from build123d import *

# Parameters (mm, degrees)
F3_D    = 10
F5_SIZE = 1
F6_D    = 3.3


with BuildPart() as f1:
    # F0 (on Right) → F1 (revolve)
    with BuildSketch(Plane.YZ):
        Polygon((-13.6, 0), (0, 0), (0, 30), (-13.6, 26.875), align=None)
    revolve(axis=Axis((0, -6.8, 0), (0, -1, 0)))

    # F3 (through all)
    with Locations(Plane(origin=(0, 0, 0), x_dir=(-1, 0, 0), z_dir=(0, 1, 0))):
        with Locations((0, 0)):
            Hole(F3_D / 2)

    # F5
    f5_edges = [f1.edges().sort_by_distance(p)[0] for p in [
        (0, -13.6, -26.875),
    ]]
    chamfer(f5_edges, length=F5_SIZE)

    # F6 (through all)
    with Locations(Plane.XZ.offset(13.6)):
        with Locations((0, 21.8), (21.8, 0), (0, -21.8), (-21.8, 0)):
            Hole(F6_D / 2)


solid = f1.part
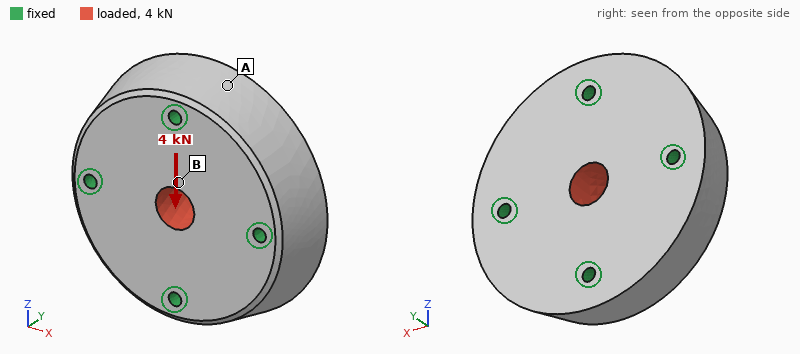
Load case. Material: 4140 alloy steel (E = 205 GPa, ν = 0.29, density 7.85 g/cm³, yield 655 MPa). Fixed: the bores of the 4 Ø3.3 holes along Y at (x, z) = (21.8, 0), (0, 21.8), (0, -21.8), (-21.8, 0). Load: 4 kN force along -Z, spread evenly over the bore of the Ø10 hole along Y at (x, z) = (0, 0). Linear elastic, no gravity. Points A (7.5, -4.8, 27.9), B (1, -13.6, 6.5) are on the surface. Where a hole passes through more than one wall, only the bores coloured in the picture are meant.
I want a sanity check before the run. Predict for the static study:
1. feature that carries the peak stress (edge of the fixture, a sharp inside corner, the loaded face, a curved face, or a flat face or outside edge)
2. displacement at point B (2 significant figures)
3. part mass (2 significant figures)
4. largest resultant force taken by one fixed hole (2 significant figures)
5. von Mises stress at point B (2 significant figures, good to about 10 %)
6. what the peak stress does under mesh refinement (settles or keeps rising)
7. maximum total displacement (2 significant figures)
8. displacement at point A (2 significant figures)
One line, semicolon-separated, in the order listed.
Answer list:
edge of the fixture; 0.66 µm; 260 g; 1.3 kN; 10 MPa; keeps rising; 0.78 µm; 0.18 µm
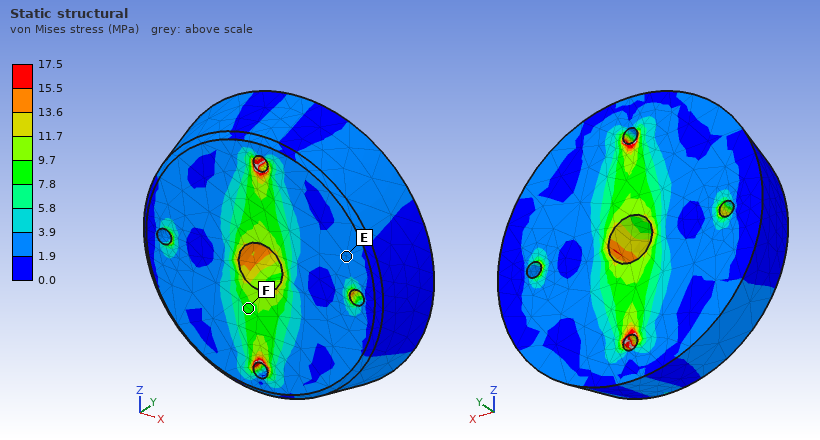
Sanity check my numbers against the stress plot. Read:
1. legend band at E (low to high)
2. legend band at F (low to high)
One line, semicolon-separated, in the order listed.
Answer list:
1.9 to 3.9 MPa; 7.8 to 9.7 MPa
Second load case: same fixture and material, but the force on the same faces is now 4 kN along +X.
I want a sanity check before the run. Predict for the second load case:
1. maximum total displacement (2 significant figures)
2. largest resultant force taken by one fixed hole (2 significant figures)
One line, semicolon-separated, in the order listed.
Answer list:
0.78 µm; 1.3 kN
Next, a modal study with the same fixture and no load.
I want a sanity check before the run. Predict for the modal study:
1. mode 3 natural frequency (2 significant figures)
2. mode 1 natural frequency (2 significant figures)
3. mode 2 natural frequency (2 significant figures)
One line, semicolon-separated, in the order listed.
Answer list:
31 kHz; 29 kHz; 30 kHz
